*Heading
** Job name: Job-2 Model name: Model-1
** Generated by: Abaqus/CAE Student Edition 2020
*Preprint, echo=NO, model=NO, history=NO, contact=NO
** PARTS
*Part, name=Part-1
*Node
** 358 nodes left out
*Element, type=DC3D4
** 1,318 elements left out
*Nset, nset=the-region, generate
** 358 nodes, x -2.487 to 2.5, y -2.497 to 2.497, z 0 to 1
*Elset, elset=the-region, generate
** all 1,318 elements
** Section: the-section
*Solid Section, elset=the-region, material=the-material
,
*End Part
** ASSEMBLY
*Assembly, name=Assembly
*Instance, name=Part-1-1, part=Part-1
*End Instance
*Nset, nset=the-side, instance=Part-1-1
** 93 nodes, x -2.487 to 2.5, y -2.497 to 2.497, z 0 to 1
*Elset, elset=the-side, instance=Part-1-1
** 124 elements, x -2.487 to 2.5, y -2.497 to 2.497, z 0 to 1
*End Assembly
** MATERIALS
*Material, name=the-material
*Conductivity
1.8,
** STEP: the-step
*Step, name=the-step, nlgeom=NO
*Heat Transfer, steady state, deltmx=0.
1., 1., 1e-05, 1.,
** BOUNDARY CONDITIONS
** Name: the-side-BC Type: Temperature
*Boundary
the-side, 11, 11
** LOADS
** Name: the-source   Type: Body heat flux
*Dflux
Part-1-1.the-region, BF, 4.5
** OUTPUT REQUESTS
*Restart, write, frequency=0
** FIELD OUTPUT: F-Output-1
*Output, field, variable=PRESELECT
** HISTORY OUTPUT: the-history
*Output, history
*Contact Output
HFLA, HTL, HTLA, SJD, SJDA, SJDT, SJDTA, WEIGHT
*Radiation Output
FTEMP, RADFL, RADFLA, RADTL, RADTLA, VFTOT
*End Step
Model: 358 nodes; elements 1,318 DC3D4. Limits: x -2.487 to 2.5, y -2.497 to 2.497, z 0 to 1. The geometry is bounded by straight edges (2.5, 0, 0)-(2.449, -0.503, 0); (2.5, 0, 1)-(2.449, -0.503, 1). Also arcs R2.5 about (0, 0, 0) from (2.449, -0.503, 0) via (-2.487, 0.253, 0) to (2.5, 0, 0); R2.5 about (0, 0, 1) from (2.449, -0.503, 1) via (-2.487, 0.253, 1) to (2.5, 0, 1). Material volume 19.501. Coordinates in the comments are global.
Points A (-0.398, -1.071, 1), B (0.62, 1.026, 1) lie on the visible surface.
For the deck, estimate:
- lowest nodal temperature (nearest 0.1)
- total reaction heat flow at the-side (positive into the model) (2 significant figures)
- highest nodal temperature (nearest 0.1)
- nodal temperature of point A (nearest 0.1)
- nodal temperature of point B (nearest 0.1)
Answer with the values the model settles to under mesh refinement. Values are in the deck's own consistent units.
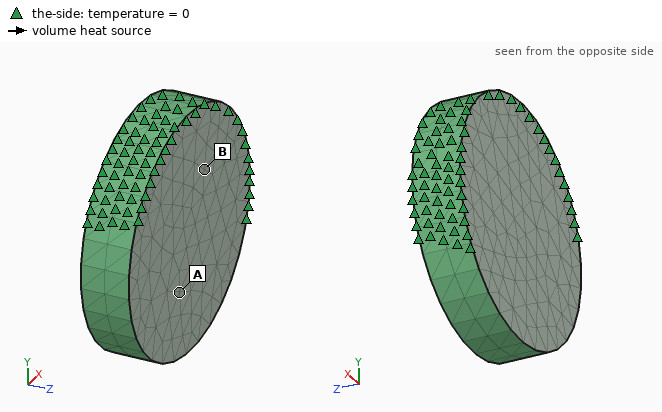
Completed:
0.0
-86
3.9
3.1
3.0
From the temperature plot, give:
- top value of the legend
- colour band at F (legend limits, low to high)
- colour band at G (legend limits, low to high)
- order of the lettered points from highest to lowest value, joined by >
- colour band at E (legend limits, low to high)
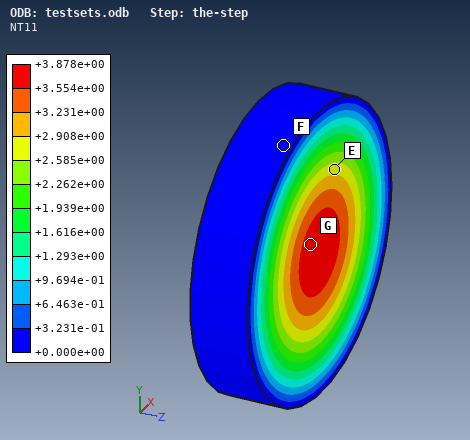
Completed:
+3.878e+00
+0.000e+00 to +3.231e-01
+3.554e+00 to +3.878e+00
G > E > F
+2.585e+00 to +2.908e+00
